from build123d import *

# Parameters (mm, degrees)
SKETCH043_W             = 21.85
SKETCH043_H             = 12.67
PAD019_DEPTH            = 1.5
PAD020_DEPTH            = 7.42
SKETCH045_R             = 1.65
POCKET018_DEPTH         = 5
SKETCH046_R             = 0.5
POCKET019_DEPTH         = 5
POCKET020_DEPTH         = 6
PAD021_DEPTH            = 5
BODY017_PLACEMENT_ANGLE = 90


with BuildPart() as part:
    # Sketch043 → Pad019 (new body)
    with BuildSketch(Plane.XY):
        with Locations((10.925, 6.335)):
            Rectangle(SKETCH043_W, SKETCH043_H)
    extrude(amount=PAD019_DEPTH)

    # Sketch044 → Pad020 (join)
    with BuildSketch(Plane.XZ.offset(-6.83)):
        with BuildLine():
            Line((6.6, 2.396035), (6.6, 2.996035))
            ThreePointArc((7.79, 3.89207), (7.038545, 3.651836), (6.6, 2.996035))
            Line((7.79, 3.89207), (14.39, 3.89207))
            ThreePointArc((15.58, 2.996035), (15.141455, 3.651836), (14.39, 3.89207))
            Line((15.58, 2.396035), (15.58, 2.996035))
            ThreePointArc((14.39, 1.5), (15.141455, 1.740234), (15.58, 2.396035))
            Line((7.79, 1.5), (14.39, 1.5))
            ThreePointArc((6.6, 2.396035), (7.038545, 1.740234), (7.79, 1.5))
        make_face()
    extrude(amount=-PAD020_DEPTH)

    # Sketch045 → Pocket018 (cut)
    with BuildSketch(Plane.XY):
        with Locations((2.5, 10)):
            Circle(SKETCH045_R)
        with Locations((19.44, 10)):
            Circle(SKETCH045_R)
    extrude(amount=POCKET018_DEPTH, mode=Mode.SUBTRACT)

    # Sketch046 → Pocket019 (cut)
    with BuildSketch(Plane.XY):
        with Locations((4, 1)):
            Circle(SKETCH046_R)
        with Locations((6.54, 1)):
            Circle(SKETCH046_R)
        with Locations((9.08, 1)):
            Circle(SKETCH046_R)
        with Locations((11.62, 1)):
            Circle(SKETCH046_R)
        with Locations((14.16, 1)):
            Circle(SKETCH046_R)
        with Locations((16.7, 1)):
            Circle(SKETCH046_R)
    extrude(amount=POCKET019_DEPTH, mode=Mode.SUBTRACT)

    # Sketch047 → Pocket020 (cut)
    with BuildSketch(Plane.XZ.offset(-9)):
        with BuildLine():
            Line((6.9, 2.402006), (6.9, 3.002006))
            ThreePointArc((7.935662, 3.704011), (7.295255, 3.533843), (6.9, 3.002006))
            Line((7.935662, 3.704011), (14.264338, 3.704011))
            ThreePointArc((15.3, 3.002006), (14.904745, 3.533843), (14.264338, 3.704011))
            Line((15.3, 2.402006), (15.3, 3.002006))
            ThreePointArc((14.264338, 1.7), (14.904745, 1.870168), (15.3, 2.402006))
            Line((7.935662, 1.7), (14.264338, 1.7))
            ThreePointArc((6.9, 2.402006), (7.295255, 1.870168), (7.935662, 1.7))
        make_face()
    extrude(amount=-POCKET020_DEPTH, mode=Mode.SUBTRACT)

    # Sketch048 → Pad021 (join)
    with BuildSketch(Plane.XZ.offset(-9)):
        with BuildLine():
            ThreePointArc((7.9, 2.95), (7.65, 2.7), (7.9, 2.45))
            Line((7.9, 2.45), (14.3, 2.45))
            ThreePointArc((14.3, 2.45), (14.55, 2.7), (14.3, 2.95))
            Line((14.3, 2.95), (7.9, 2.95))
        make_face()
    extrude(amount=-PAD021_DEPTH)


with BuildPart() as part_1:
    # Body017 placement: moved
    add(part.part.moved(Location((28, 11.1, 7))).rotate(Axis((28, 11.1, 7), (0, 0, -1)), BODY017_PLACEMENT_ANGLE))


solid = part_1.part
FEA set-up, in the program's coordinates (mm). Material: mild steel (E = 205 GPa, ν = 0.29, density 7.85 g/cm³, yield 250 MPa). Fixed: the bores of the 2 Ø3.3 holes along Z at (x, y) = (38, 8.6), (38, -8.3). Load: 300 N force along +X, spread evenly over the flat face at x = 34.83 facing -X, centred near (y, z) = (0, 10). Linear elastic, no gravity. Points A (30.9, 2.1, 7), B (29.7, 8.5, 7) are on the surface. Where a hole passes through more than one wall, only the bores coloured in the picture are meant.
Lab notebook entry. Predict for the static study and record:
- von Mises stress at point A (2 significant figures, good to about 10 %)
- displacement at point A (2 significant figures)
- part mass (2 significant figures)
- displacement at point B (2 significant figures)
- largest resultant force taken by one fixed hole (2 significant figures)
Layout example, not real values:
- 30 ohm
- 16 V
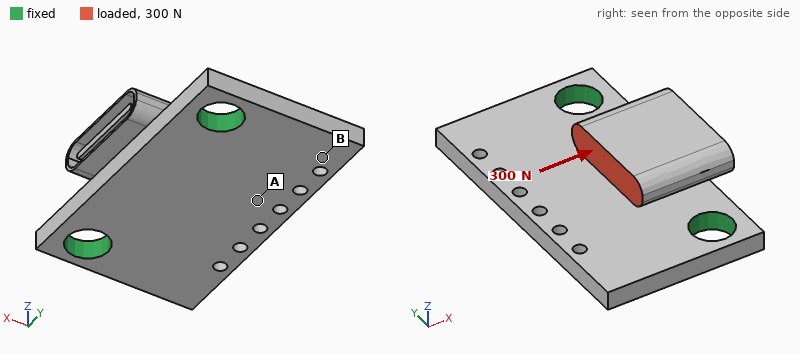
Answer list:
- 31 MPa
- 7.9 µm
- 3.7 g
- 5.4 µm
- 160 N
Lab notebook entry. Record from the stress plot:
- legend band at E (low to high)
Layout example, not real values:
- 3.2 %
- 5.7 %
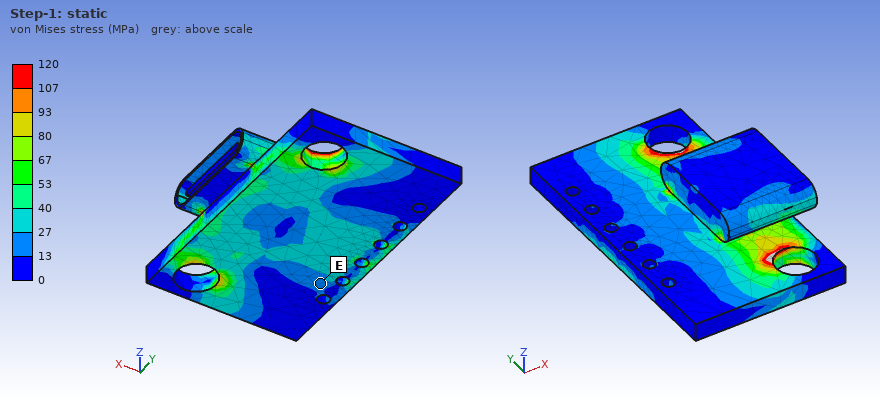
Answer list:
- 13 to 27 MPa
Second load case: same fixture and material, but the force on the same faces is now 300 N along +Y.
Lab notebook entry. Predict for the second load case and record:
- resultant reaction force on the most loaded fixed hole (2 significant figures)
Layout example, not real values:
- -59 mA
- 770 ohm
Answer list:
- 170 N
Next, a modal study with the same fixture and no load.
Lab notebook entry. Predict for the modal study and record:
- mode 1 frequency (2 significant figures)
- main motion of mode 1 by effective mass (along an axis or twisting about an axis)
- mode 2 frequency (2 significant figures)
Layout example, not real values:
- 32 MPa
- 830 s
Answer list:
- 13 kHz
- along Z
- 15 kHz
